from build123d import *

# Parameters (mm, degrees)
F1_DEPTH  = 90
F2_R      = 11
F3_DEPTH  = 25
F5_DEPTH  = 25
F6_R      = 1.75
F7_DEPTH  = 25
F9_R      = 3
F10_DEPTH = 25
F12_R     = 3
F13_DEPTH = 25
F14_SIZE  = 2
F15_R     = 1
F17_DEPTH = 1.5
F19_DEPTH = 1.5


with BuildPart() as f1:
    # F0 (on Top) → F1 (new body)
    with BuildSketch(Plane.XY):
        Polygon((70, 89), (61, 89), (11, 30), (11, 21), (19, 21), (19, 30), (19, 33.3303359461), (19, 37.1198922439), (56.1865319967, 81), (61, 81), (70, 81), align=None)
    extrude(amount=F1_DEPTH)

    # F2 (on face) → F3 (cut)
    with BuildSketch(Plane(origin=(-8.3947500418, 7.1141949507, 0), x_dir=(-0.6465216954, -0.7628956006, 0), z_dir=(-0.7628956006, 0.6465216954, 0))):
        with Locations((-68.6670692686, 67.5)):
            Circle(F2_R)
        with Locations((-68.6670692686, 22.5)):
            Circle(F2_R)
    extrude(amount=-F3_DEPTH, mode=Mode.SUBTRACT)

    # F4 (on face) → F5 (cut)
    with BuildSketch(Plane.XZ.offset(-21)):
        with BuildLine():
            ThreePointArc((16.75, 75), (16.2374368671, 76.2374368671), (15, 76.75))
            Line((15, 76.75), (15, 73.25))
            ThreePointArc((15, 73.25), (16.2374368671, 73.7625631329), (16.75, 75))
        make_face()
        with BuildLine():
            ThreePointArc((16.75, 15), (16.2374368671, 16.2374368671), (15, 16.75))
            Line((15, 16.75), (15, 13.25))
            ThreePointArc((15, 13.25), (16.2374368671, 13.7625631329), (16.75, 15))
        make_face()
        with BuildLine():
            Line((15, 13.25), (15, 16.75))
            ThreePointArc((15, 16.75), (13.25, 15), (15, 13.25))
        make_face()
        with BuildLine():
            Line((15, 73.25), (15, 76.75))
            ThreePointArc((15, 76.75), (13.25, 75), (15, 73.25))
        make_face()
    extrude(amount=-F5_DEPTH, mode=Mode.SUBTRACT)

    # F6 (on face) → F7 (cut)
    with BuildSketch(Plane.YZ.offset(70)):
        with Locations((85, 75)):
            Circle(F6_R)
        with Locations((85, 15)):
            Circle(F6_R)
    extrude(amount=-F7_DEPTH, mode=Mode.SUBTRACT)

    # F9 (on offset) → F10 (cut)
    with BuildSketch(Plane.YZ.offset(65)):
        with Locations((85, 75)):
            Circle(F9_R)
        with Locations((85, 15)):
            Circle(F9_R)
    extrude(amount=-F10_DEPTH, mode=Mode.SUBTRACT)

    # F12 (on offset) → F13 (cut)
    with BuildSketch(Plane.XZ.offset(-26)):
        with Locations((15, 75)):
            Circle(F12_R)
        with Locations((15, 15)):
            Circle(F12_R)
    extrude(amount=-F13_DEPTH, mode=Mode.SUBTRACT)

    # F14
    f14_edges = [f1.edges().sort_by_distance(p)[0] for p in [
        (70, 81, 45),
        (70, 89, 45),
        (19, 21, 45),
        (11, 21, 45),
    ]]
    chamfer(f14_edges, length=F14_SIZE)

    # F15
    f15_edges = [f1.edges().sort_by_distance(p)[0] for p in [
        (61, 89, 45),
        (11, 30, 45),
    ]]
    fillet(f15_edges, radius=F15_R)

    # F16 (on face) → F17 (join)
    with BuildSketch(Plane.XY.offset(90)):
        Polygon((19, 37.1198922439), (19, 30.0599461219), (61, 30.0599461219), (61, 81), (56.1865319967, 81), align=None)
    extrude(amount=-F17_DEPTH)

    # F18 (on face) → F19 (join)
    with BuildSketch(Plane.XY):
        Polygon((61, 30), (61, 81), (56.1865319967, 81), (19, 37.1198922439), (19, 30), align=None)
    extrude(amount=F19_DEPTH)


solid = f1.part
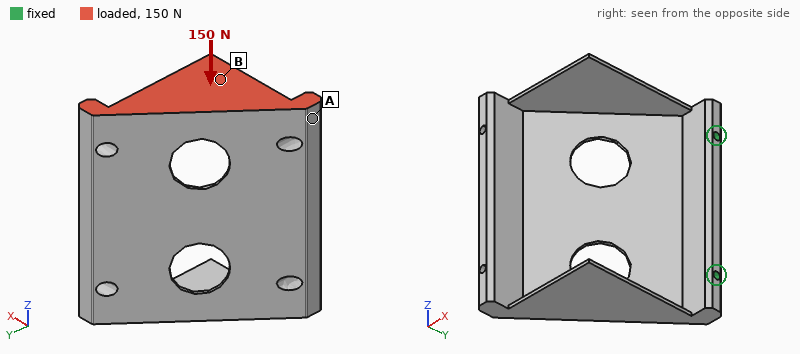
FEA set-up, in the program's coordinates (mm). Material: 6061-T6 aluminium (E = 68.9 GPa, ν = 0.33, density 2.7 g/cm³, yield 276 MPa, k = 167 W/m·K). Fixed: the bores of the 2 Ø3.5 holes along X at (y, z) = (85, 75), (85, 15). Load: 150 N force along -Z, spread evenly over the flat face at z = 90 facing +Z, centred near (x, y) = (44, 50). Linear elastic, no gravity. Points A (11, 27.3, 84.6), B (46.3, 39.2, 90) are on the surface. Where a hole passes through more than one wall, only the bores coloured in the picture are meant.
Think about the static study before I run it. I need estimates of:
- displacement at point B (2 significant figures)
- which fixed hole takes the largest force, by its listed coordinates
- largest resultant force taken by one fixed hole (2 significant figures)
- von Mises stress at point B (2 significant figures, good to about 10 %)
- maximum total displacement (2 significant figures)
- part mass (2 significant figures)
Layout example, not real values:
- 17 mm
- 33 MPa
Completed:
- 0.35 mm
- (85, 75)
- 150 N
- 19 MPa
- 0.73 mm
- 74 g
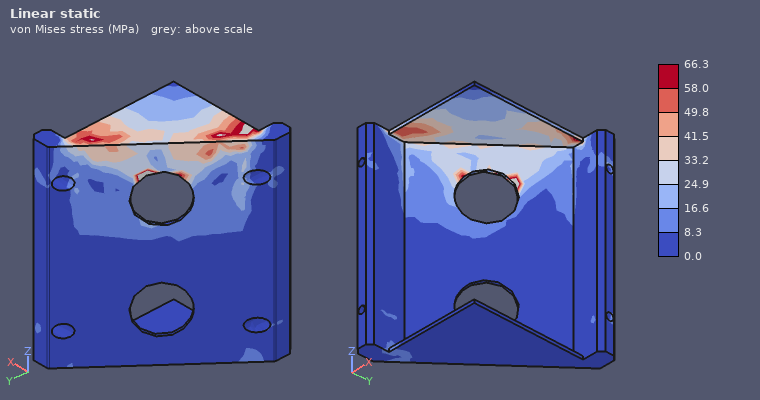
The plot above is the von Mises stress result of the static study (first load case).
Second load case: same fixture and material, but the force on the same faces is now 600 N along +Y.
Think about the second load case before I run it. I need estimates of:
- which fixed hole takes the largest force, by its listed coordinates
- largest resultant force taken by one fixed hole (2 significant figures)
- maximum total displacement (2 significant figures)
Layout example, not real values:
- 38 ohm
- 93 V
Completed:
- (85, 75)
- 760 N
- 1.3 mm
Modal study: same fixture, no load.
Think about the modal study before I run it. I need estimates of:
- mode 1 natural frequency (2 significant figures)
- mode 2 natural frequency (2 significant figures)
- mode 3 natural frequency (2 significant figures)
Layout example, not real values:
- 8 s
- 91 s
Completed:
- 360 Hz
- 740 Hz
- 1300 Hz
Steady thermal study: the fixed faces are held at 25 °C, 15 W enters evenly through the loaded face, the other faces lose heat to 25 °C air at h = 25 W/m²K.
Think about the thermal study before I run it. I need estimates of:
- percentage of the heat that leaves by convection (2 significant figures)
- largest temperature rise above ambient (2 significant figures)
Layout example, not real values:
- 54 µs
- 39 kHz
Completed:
- 36 %
- 37 K
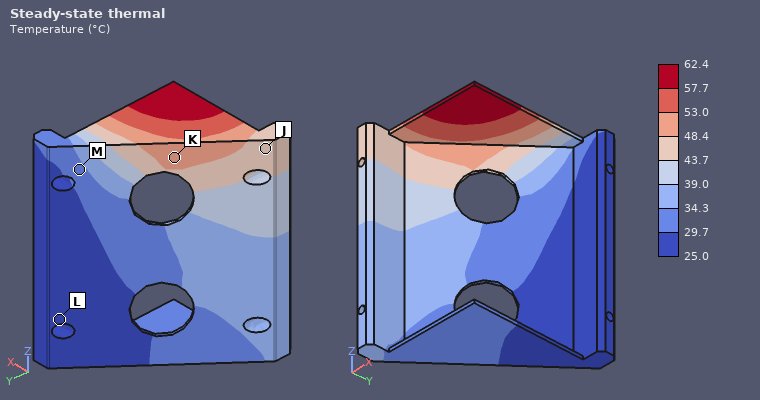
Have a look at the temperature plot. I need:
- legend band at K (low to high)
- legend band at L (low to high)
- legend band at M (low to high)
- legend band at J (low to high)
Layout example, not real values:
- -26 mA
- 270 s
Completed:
- 48.4 to 53.0 °C
- 25.0 to 29.7 °C
- 29.7 to 34.3 °C
- 43.7 to 48.4 °C
